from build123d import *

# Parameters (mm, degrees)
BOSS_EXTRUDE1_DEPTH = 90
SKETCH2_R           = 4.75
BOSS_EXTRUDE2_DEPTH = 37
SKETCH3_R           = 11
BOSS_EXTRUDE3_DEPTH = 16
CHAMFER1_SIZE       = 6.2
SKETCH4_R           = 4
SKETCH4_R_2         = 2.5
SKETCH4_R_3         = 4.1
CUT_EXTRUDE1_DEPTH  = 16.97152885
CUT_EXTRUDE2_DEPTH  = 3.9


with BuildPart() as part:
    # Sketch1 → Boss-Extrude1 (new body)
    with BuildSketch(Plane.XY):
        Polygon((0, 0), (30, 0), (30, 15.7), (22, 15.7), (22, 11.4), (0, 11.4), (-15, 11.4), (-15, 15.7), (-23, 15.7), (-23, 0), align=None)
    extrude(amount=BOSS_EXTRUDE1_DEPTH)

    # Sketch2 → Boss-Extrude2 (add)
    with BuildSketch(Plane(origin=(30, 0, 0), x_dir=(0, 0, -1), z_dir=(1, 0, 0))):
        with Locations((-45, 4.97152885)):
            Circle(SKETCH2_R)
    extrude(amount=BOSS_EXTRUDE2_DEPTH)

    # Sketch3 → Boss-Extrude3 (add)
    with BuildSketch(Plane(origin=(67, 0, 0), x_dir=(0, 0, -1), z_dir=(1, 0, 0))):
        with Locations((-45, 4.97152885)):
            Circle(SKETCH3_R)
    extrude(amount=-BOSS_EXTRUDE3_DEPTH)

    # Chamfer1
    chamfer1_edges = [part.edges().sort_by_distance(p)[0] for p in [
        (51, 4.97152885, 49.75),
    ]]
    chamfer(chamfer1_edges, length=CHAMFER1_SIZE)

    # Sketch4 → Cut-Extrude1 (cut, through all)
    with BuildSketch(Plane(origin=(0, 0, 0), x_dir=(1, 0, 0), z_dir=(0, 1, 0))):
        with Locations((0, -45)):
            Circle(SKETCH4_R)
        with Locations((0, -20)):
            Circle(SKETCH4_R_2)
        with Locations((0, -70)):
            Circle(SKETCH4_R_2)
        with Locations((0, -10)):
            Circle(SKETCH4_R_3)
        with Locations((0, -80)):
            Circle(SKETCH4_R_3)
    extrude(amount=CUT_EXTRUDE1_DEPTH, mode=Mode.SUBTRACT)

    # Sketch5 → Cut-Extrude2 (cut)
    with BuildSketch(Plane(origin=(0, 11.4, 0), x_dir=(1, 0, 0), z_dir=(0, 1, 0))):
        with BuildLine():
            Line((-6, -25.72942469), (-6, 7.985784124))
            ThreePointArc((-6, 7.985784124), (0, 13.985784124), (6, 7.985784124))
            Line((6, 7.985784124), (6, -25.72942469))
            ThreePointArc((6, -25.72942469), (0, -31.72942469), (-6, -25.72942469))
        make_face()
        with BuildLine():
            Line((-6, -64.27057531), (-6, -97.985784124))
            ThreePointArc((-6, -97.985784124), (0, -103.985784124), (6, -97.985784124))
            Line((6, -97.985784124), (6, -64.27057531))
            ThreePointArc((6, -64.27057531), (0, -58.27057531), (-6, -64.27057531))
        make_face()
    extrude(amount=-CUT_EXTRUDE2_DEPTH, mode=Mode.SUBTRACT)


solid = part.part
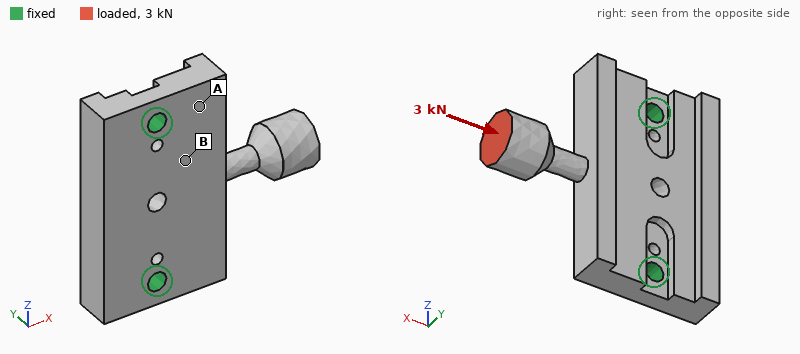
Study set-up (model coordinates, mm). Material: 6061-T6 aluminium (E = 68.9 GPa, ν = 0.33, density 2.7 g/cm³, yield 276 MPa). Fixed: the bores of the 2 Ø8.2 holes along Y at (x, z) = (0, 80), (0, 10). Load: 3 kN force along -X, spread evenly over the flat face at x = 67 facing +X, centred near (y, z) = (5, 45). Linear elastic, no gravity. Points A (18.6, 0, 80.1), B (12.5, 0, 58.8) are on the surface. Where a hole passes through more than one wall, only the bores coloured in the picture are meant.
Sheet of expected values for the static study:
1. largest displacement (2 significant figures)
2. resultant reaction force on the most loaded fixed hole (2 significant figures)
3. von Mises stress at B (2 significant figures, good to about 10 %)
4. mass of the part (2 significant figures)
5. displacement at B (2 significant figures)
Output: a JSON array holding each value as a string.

["24 µm", "1.6 kN", "8.2 MPa", "170 g", "4.5 µm"]
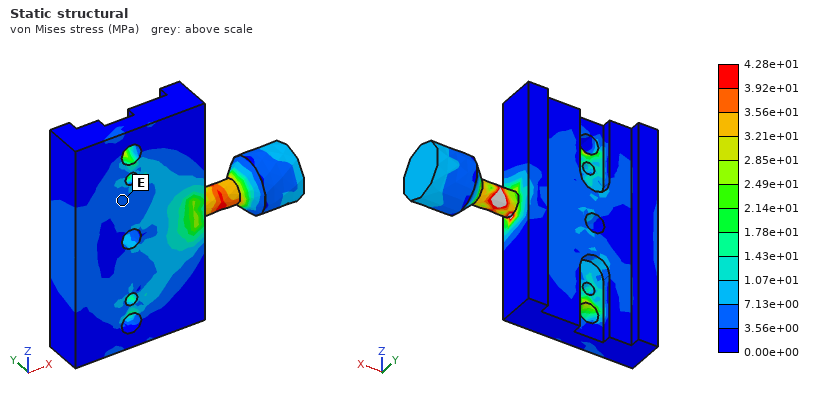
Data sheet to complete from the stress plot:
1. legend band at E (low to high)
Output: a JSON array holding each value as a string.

["3.56e+00 to 7.13e+00 MPa"]
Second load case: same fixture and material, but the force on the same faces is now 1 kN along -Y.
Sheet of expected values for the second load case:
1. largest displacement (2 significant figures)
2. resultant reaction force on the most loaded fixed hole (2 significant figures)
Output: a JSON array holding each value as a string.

["0.98 mm", "640 N"]
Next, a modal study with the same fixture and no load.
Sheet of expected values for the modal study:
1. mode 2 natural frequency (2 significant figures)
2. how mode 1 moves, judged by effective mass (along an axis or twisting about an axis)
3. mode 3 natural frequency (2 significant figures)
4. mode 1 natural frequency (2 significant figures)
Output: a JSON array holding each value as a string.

["1900 Hz", "along Y", "4800 Hz", "1500 Hz"]
